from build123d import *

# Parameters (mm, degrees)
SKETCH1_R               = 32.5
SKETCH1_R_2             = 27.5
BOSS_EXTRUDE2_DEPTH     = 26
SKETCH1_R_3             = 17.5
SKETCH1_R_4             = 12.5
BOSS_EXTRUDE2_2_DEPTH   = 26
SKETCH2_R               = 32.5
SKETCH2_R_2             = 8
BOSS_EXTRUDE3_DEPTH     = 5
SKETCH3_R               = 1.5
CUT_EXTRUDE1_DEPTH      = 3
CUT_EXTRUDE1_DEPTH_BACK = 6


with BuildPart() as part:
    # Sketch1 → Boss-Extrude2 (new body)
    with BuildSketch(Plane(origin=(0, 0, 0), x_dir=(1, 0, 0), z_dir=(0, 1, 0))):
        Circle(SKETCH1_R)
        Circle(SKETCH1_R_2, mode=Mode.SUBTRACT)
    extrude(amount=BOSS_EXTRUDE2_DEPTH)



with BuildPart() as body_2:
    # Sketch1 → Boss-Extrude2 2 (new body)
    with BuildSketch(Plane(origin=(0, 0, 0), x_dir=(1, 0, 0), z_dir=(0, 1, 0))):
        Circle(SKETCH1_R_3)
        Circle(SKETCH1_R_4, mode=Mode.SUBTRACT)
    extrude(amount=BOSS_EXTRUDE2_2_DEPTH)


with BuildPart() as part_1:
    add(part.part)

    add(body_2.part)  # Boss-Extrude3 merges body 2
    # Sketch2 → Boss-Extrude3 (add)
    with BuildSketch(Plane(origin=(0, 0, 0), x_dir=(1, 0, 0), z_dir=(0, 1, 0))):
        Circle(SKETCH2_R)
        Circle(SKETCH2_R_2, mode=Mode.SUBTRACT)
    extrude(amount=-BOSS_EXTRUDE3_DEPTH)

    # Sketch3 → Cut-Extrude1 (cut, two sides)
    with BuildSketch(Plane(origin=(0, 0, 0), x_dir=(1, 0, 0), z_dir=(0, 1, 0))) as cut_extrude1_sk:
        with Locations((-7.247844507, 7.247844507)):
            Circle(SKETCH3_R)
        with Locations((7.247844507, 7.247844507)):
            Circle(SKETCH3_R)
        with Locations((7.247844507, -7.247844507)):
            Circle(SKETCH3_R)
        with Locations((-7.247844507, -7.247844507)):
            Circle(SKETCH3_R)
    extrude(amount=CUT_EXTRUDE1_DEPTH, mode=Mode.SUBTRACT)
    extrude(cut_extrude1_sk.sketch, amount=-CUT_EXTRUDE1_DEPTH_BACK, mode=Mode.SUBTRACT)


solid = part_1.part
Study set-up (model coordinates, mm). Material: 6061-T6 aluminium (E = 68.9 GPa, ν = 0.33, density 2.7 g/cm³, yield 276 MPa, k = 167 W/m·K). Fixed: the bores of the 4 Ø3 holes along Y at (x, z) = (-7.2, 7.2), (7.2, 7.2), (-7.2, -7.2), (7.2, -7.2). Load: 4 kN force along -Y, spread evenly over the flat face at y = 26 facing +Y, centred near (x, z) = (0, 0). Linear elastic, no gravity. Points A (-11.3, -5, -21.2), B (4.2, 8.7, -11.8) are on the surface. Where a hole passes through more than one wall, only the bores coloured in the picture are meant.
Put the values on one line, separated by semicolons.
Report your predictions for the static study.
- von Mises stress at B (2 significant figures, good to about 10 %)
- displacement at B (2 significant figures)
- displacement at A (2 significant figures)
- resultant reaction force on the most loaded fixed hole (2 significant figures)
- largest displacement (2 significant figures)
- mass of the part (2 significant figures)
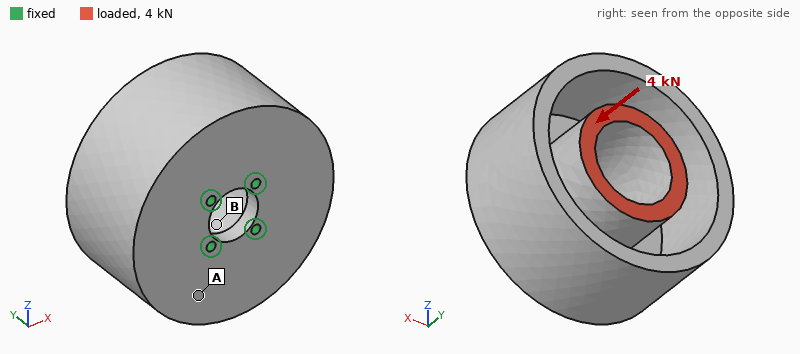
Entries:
11 MPa; 5.3 µm; 5.9 µm; 1.0 kN; 7.3 µm; 140 g
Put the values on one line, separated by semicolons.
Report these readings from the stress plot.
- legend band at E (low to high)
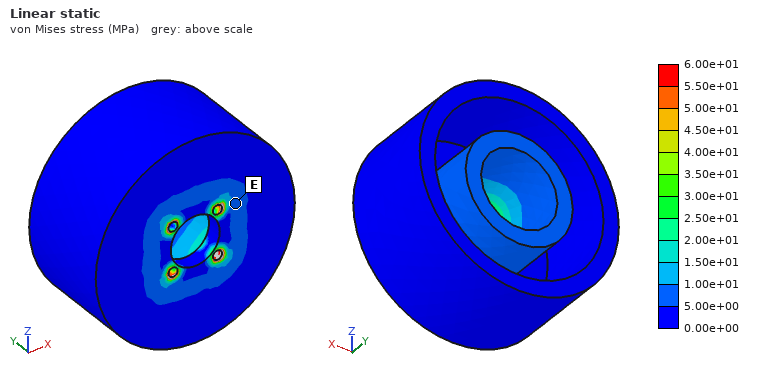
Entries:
5.00e+00 to 1.00e+01 MPa
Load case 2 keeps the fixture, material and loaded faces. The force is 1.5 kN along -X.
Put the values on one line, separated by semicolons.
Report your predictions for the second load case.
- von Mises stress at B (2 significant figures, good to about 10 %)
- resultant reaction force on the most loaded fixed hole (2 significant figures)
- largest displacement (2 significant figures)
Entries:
15 MPa; 1.1 kN; 32 µm
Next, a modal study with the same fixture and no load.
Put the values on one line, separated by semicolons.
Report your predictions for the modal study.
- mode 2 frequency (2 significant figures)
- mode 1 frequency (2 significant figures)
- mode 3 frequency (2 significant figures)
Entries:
3300 Hz; 3300 Hz; 5300 Hz
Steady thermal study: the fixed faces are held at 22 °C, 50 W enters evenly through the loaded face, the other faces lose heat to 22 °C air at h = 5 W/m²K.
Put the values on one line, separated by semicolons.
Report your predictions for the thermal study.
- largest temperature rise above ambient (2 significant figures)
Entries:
21 K
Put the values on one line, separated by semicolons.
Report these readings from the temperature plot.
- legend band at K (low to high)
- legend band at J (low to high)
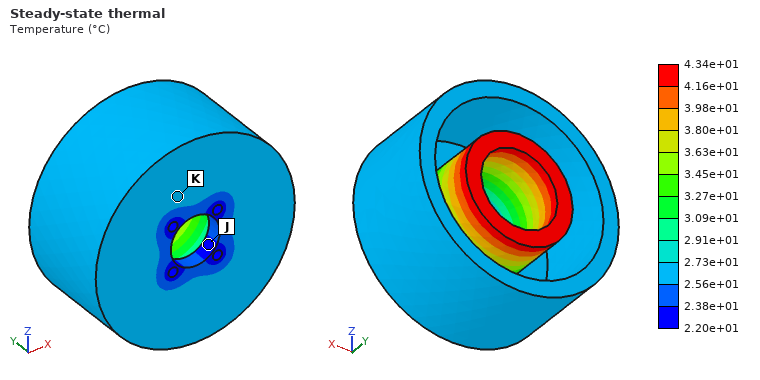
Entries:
2.56e+01 to 2.73e+01 °C; 2.20e+01 to 2.38e+01 °C
